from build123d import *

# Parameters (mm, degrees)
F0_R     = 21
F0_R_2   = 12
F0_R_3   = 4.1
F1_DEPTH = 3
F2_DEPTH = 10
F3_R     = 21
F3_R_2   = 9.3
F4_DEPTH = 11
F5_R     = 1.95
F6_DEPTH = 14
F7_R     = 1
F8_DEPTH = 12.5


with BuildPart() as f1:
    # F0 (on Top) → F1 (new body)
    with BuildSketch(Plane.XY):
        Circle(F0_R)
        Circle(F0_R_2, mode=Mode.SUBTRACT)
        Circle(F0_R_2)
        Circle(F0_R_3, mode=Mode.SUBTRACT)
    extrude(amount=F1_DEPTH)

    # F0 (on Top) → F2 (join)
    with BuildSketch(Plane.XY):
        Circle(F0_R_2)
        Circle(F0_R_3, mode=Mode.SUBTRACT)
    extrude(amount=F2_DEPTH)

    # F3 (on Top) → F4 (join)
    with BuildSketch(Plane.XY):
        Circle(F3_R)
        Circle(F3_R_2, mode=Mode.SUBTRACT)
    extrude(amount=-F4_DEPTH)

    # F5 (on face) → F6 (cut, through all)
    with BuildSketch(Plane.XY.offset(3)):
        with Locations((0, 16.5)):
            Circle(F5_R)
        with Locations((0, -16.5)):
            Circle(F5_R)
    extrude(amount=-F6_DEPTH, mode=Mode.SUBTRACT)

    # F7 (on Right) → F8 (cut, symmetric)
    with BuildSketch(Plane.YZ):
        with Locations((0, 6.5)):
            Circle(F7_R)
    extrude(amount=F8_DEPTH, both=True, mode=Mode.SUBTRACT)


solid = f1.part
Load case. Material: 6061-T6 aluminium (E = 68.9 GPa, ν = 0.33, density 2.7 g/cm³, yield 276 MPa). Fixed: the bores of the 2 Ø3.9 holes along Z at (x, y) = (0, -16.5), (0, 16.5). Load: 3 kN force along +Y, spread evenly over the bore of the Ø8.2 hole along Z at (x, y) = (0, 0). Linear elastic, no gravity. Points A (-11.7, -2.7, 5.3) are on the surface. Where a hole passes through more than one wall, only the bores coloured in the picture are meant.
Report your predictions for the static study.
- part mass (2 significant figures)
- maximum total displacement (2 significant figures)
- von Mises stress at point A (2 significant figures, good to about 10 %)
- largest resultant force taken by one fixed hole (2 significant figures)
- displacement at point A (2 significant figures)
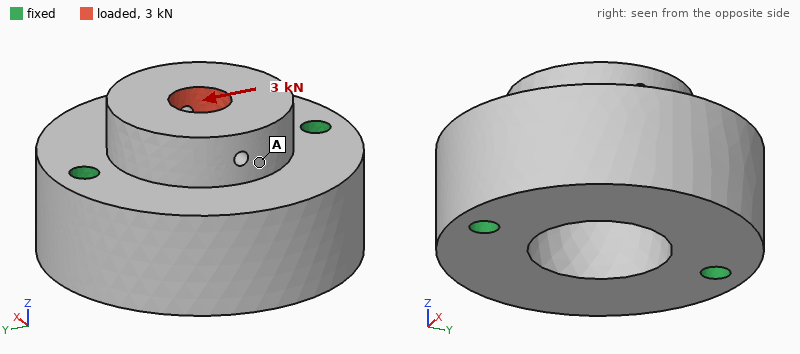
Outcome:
50 g
5.3 µm
5.2 MPa
1.6 kN
2.5 µm
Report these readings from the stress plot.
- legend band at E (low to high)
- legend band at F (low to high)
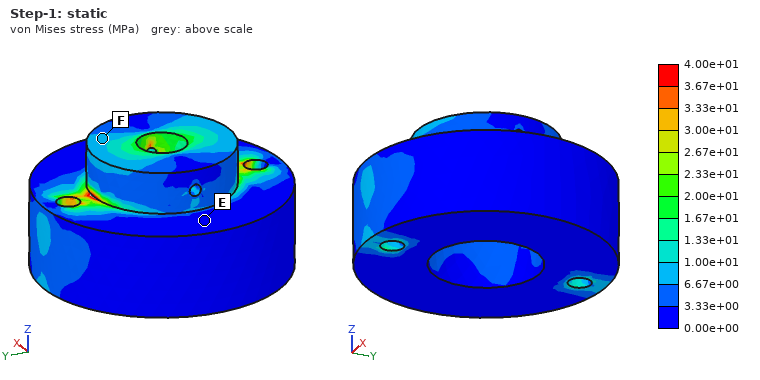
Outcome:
0.00e+00 to 3.33e+00 MPa
6.67e+00 to 1.00e+01 MPa
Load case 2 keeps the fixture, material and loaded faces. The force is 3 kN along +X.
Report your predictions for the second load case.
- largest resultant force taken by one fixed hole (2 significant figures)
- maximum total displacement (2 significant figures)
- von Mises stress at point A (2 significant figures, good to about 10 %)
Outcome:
1.5 kN
11 µm
6.6 MPa
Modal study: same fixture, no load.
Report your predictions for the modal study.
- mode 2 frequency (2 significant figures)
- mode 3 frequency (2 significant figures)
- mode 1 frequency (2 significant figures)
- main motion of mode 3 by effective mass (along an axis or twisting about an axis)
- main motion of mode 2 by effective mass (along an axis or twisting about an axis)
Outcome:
21 kHz
30 kHz
16 kHz
twisting about Z
along Z
